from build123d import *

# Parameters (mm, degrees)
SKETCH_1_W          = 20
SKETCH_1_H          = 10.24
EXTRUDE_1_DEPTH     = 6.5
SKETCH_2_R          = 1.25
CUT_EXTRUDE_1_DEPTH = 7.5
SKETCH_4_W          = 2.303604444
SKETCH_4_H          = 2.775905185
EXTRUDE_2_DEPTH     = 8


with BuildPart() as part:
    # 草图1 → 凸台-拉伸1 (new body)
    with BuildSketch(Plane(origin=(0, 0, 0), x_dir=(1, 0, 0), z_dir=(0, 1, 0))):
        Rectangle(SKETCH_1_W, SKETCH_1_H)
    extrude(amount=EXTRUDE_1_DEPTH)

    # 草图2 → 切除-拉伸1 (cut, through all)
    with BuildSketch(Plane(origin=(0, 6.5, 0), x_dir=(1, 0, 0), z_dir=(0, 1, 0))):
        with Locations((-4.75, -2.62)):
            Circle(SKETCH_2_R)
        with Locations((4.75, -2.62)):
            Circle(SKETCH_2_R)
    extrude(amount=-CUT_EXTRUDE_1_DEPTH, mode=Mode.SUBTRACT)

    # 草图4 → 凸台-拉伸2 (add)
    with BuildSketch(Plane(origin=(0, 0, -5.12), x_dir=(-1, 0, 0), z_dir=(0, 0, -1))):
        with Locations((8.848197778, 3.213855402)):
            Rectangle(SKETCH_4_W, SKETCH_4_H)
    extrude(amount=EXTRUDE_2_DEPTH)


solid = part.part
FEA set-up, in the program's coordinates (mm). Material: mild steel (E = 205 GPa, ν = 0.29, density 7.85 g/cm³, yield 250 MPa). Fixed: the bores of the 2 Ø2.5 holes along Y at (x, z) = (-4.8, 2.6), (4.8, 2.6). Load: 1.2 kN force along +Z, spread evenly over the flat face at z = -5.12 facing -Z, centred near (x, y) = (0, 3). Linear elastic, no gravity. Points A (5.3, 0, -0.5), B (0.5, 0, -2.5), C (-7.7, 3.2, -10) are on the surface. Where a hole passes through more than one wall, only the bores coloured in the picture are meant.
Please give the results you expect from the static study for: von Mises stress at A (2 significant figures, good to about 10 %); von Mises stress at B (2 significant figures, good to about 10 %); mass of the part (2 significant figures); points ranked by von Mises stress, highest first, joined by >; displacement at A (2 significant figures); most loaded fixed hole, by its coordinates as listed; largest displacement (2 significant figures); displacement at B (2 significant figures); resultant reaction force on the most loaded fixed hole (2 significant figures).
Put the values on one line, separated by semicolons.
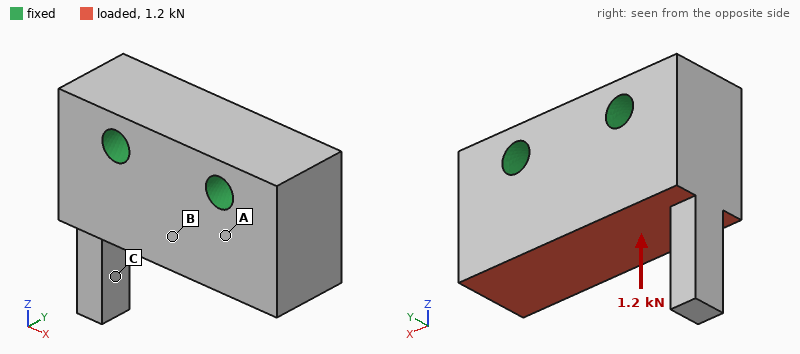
15 MPa; 8.4 MPa; 10 g; A > B > C; 0.21 µm; (4.8, 2.6); 0.67 µm; 0.29 µm; 650 N
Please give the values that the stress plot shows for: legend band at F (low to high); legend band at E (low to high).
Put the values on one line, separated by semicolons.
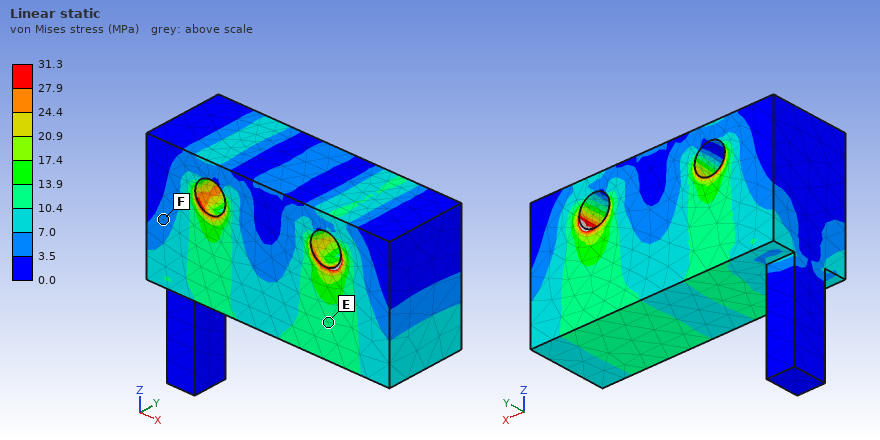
3.5 to 7.0 MPa; 10.4 to 13.9 MPa
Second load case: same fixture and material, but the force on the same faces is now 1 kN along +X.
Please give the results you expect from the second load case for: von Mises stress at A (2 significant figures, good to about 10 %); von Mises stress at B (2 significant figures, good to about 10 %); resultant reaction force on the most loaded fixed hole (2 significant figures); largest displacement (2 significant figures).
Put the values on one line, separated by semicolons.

15 MPa; 25 MPa; 790 N; 3.2 µm
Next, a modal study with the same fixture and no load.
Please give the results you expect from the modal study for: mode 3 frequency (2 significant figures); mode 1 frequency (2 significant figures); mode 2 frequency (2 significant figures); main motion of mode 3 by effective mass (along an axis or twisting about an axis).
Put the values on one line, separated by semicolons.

59 kHz; 22 kHz; 25 kHz; along Y
